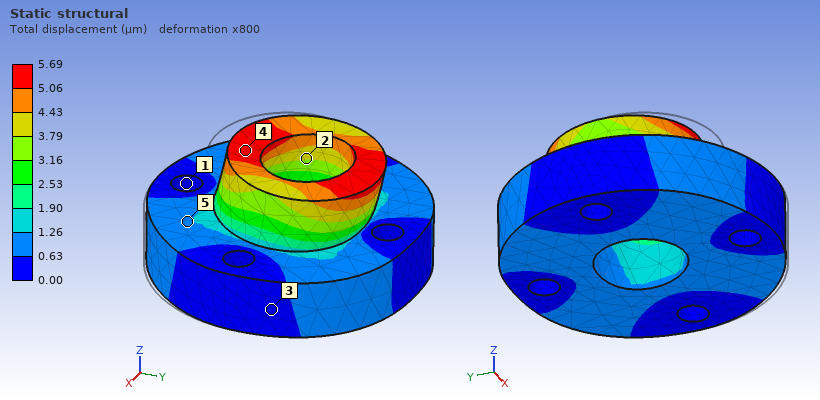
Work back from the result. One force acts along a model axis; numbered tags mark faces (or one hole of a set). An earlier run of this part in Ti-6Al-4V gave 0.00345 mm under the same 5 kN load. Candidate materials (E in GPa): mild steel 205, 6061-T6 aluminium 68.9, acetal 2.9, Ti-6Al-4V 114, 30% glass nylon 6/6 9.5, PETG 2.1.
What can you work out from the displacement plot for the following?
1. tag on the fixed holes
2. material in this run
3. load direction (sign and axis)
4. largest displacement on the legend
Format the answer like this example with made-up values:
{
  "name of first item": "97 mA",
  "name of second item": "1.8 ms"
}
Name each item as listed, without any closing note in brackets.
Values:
{
  "tag on the fixed holes": "1",
  "material in this run": "6061-T6 aluminium",
  "load direction": "+Y",
  "largest displacement on the legend": "5.69 µm"
}
